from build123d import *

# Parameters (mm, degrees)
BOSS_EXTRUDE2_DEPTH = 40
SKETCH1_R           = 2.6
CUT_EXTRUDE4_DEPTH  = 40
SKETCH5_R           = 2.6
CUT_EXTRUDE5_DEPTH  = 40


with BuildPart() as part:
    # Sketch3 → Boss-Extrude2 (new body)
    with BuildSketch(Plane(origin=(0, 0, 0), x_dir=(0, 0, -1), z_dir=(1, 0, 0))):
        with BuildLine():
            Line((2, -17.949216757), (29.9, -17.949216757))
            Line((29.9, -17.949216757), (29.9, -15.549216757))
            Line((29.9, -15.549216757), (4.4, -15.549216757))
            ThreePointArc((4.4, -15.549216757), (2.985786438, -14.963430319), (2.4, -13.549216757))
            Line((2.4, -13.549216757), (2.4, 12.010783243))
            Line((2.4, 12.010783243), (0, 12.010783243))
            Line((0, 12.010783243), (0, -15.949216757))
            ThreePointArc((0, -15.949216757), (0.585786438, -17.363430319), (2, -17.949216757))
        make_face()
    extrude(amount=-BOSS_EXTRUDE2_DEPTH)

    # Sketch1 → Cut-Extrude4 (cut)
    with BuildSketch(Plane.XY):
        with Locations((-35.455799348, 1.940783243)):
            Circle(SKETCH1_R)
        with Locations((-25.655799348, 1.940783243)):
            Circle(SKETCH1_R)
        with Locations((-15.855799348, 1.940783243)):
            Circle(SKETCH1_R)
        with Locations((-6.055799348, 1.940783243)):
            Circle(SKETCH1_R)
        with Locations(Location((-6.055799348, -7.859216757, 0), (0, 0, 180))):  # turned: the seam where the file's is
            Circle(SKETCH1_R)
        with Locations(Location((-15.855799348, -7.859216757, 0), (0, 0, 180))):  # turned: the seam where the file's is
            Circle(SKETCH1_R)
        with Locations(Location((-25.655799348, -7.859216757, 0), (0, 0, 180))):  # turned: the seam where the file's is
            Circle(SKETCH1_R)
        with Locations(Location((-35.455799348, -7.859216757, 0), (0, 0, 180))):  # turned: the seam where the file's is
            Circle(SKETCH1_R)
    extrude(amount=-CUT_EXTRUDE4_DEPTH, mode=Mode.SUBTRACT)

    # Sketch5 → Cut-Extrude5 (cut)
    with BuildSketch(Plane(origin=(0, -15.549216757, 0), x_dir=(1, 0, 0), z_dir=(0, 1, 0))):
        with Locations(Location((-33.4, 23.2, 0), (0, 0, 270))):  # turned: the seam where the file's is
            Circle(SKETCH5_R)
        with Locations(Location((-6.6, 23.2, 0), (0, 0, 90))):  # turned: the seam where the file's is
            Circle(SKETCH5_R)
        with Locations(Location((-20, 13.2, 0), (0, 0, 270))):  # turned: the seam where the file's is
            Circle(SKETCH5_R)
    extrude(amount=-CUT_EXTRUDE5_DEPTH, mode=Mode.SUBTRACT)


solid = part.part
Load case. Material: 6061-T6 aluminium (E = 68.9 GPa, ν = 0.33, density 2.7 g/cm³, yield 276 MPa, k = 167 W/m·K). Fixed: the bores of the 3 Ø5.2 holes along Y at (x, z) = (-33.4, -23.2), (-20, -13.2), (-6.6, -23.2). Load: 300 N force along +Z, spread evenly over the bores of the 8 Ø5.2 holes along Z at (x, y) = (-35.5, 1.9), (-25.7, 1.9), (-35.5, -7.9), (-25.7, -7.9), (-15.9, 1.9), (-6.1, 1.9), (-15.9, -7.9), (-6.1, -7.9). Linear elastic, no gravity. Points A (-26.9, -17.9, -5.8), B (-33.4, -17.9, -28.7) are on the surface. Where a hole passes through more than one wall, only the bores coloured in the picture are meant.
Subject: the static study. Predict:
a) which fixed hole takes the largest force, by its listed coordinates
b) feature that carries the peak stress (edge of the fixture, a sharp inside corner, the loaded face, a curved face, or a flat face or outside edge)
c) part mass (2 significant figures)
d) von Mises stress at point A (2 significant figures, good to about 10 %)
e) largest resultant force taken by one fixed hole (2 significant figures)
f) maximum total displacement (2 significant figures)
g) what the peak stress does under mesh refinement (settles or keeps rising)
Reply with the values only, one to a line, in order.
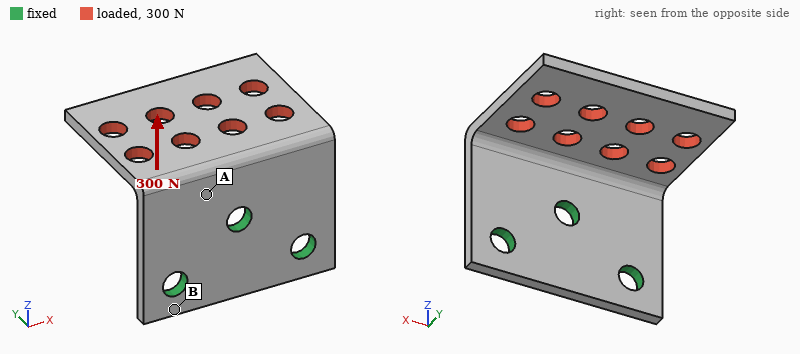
(-20, -13.2)
edge of the fixture
13 g
97 MPa
230 N
0.63 mm
keeps rising
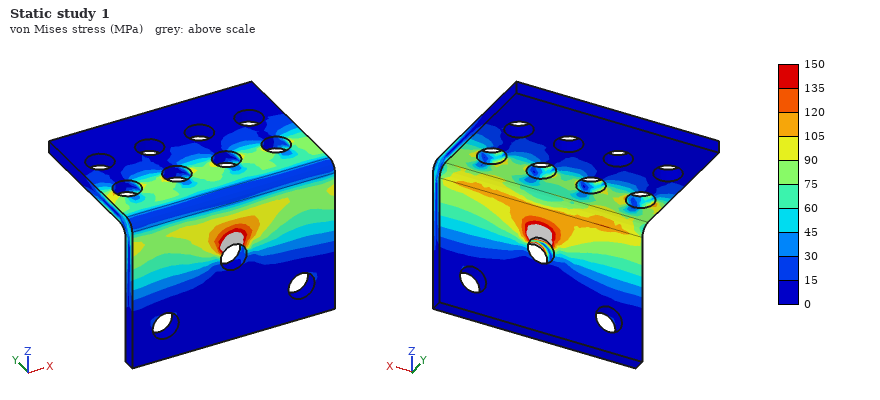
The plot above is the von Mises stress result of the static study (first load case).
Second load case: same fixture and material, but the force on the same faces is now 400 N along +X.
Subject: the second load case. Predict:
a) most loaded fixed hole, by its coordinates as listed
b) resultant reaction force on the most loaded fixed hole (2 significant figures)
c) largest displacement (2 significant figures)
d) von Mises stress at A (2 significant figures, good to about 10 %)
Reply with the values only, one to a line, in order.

(-20, -13.2)
360 N
0.29 mm
39 MPa
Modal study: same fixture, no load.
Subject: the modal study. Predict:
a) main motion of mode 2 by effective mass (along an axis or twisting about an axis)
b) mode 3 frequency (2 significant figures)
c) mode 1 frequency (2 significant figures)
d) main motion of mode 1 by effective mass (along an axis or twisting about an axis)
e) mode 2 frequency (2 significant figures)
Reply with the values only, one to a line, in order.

along X
4100 Hz
1500 Hz
along Z
2400 Hz
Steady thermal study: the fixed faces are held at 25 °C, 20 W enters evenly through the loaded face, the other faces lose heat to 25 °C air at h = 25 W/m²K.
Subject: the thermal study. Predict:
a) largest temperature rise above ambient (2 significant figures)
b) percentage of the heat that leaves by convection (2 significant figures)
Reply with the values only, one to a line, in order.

37 K
9.6 %
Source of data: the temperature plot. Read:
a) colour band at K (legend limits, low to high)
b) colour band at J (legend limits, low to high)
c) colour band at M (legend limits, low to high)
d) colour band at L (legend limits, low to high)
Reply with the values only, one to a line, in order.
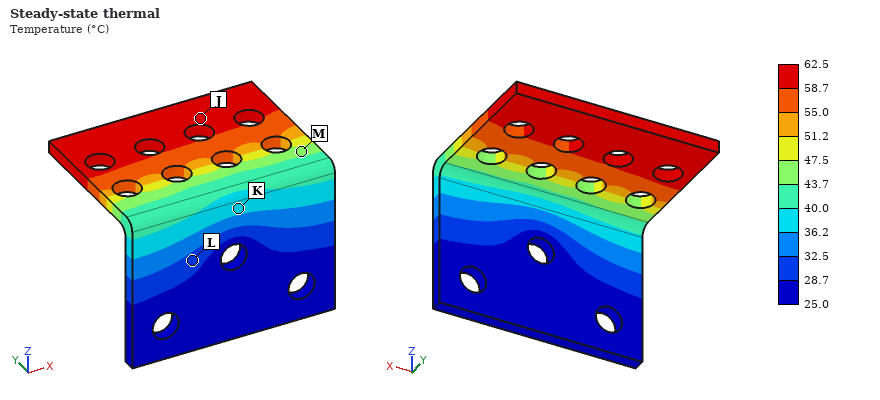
36.2 to 40.0 °C
58.7 to 62.5 °C
43.7 to 47.5 °C
28.7 to 32.5 °C
